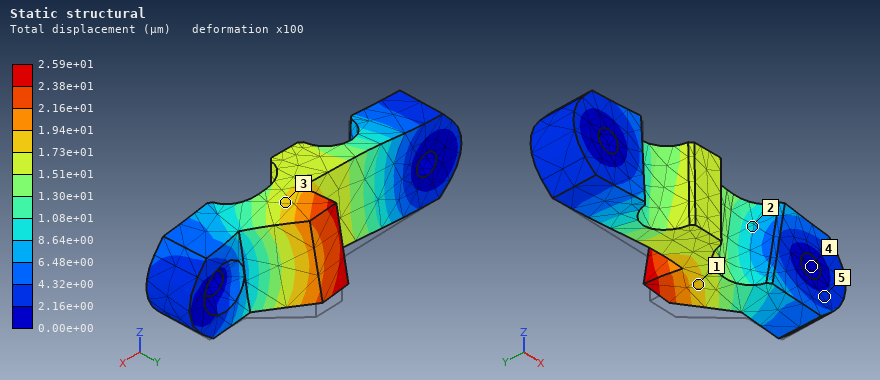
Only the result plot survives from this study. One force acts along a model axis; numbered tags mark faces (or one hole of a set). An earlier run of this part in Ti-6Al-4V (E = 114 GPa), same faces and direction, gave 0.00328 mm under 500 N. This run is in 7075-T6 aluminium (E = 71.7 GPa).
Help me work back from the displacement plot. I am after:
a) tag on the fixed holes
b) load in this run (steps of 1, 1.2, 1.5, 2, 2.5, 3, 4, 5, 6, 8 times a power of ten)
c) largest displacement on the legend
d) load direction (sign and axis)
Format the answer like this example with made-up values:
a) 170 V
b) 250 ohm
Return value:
a) 4
b) 2.5 kN
c) 2.59e+01 µm
d) +Z
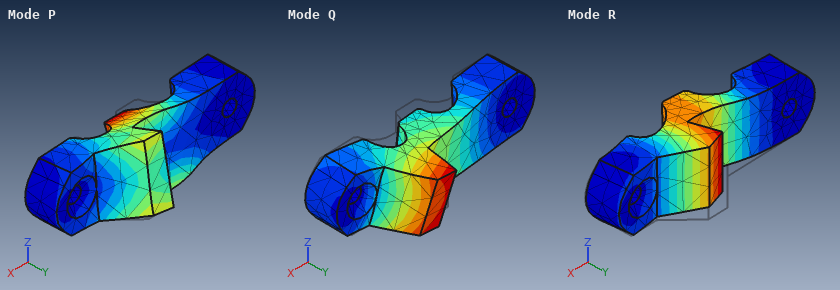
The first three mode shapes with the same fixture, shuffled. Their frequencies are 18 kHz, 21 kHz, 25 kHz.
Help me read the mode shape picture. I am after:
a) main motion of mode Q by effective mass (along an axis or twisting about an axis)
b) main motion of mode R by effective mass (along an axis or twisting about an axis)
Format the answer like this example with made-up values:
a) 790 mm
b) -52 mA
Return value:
a) along Z
b) along Y
